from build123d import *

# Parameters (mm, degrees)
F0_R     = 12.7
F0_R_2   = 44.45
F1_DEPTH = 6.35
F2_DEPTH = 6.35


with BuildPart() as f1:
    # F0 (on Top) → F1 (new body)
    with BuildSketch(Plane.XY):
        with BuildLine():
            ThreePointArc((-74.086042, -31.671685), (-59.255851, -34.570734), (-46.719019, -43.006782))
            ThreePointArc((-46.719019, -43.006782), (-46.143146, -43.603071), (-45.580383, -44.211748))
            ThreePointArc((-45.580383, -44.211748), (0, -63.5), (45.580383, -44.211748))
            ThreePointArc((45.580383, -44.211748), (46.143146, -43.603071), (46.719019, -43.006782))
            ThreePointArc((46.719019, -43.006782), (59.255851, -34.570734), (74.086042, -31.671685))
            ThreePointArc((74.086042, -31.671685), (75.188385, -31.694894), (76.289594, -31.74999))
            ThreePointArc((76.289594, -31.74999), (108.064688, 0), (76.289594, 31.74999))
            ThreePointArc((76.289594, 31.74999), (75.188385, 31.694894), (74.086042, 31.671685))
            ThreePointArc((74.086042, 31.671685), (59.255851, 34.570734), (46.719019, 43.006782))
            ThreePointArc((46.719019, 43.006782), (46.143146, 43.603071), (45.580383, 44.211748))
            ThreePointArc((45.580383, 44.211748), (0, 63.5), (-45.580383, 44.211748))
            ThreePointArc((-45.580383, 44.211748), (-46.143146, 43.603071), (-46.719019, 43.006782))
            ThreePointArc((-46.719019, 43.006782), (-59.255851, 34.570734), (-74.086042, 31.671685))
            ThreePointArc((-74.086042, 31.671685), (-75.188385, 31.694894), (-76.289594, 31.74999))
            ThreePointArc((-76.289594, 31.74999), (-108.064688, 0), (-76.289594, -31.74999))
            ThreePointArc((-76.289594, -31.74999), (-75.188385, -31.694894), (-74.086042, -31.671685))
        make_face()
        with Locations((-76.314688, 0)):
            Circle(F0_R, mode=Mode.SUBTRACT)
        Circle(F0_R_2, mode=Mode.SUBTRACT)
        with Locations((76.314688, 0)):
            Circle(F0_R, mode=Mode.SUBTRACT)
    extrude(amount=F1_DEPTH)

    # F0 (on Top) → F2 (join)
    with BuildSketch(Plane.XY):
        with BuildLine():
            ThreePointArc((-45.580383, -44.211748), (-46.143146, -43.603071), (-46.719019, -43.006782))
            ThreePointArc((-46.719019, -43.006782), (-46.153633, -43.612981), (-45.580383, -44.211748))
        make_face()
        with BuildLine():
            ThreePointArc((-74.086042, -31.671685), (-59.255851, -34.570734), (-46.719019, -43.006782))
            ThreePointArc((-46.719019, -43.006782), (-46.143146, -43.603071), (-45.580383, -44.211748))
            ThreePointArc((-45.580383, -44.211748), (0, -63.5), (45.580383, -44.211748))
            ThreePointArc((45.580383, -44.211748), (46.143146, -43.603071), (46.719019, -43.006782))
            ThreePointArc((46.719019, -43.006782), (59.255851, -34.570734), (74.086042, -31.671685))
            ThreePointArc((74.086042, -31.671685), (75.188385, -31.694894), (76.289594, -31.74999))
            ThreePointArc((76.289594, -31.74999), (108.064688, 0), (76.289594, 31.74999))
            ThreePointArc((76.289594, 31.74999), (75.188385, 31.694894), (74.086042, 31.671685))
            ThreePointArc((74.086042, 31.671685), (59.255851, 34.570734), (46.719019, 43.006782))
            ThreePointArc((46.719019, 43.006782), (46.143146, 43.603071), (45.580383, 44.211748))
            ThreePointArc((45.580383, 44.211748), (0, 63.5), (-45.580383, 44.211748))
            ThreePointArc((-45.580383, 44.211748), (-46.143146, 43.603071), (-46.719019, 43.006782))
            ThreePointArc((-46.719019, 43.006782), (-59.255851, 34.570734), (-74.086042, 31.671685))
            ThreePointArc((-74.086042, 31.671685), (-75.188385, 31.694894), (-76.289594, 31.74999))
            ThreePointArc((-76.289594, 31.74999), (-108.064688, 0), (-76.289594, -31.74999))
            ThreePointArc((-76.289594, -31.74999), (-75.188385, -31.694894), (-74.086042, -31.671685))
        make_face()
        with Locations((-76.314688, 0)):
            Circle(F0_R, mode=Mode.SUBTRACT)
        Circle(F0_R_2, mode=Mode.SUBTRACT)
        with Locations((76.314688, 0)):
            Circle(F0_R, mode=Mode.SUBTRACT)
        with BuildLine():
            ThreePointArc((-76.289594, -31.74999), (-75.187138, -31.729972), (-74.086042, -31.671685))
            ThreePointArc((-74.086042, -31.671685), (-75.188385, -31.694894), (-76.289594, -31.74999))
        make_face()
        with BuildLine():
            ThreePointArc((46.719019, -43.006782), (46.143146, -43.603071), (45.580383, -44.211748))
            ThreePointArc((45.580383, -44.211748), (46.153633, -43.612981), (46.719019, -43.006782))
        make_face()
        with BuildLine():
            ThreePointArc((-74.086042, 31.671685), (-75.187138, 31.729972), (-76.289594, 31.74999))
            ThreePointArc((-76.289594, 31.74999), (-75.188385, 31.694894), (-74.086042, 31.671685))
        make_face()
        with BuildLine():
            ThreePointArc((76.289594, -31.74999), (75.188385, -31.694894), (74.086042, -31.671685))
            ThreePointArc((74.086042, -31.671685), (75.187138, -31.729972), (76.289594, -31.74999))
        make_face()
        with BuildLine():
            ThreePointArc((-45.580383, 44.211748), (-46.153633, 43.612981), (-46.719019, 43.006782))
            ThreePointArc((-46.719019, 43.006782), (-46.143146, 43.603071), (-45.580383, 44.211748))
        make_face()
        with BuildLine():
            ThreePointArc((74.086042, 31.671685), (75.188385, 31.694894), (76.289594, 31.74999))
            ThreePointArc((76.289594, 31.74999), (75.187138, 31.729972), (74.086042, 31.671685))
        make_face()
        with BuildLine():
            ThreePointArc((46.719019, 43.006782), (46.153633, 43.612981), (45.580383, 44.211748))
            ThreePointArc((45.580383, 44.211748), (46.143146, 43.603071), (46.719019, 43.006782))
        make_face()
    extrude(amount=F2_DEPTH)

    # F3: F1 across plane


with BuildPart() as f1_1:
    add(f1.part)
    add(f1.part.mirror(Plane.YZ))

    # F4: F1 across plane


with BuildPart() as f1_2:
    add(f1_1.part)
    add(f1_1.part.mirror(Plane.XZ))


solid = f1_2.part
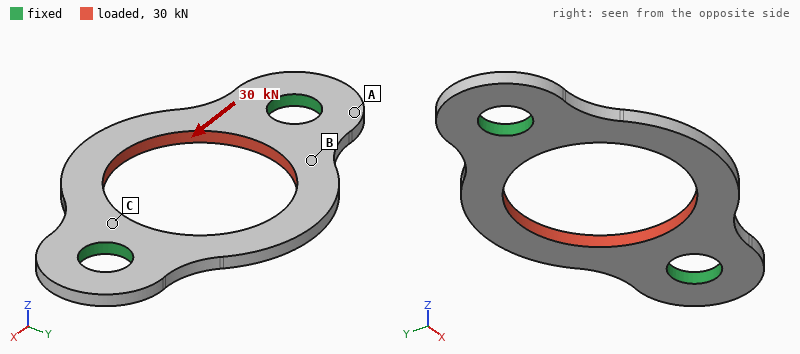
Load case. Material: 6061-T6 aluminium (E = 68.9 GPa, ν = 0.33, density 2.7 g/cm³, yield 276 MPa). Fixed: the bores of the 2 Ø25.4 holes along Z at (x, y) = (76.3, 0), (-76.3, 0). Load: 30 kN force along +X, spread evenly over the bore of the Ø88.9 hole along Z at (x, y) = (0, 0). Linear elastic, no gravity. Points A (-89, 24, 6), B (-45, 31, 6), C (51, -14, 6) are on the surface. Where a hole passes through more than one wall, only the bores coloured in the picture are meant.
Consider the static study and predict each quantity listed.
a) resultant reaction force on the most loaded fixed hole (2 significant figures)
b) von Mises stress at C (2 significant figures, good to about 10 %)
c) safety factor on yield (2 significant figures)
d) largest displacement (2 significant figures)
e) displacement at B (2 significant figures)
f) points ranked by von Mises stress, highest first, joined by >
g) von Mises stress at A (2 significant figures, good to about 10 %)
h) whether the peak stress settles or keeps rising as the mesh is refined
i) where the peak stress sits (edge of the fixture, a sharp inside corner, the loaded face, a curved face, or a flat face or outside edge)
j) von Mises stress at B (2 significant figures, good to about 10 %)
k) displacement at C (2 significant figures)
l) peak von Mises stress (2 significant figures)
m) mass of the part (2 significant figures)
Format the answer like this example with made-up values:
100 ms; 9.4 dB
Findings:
15 kN; 36 MPa; 2.8; 80 µm; 42 µm; B > C > A; 19 MPa; settles; the loaded face; 56 MPa; 12 µm; 97 MPa; 180 g
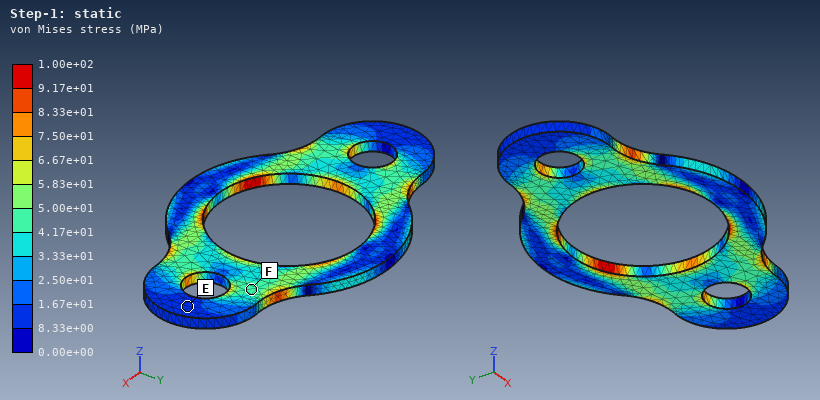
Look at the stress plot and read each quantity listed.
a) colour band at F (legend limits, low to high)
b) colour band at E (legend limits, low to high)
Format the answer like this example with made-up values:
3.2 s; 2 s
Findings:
4.17e+01 to 5.00e+01 MPa; 8.33e+00 to 1.67e+01 MPa
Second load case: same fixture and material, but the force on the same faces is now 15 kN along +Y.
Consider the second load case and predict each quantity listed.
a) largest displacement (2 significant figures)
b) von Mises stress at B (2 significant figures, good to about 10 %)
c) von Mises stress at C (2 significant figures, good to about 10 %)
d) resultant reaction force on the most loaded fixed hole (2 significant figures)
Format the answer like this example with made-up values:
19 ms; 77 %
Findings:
47 µm; 25 MPa; 31 MPa; 7.5 kN
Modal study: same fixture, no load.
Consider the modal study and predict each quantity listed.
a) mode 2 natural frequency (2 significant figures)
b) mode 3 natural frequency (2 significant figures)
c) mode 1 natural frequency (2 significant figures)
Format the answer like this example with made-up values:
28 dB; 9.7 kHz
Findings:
1200 Hz; 3200 Hz; 1200 Hz
